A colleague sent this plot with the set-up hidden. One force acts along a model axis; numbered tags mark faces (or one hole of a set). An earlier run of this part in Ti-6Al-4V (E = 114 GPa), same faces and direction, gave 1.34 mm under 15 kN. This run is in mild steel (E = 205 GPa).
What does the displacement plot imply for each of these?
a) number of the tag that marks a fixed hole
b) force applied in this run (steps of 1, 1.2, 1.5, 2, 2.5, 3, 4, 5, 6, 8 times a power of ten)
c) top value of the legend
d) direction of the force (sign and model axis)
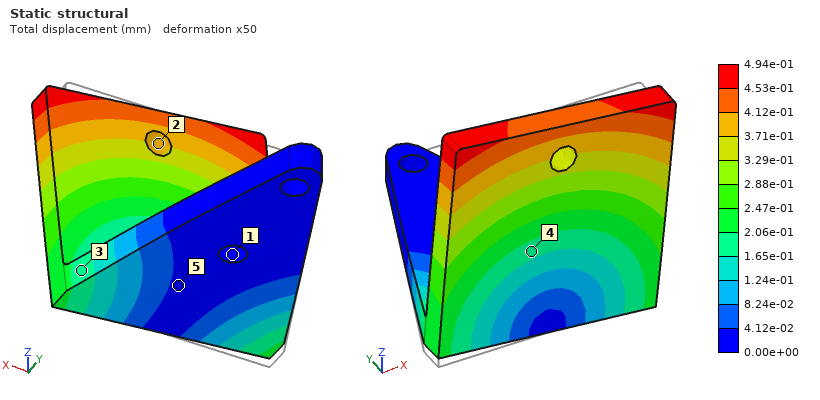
1
10 kN
4.94e-01 mm
+X
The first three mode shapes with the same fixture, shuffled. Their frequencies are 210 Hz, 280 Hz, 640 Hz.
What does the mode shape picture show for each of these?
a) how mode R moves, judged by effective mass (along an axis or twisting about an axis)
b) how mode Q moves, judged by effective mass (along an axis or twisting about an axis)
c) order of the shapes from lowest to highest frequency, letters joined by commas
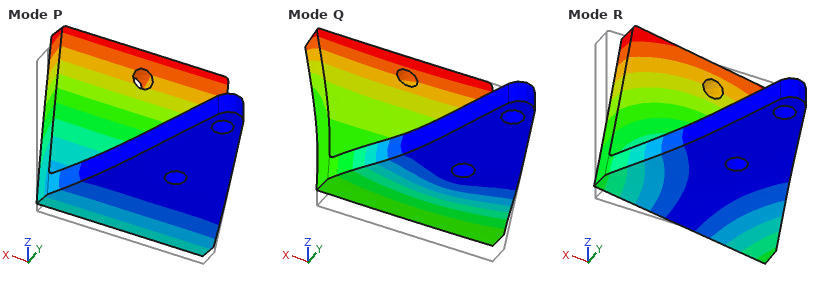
along X
along Z
P, R, Q
